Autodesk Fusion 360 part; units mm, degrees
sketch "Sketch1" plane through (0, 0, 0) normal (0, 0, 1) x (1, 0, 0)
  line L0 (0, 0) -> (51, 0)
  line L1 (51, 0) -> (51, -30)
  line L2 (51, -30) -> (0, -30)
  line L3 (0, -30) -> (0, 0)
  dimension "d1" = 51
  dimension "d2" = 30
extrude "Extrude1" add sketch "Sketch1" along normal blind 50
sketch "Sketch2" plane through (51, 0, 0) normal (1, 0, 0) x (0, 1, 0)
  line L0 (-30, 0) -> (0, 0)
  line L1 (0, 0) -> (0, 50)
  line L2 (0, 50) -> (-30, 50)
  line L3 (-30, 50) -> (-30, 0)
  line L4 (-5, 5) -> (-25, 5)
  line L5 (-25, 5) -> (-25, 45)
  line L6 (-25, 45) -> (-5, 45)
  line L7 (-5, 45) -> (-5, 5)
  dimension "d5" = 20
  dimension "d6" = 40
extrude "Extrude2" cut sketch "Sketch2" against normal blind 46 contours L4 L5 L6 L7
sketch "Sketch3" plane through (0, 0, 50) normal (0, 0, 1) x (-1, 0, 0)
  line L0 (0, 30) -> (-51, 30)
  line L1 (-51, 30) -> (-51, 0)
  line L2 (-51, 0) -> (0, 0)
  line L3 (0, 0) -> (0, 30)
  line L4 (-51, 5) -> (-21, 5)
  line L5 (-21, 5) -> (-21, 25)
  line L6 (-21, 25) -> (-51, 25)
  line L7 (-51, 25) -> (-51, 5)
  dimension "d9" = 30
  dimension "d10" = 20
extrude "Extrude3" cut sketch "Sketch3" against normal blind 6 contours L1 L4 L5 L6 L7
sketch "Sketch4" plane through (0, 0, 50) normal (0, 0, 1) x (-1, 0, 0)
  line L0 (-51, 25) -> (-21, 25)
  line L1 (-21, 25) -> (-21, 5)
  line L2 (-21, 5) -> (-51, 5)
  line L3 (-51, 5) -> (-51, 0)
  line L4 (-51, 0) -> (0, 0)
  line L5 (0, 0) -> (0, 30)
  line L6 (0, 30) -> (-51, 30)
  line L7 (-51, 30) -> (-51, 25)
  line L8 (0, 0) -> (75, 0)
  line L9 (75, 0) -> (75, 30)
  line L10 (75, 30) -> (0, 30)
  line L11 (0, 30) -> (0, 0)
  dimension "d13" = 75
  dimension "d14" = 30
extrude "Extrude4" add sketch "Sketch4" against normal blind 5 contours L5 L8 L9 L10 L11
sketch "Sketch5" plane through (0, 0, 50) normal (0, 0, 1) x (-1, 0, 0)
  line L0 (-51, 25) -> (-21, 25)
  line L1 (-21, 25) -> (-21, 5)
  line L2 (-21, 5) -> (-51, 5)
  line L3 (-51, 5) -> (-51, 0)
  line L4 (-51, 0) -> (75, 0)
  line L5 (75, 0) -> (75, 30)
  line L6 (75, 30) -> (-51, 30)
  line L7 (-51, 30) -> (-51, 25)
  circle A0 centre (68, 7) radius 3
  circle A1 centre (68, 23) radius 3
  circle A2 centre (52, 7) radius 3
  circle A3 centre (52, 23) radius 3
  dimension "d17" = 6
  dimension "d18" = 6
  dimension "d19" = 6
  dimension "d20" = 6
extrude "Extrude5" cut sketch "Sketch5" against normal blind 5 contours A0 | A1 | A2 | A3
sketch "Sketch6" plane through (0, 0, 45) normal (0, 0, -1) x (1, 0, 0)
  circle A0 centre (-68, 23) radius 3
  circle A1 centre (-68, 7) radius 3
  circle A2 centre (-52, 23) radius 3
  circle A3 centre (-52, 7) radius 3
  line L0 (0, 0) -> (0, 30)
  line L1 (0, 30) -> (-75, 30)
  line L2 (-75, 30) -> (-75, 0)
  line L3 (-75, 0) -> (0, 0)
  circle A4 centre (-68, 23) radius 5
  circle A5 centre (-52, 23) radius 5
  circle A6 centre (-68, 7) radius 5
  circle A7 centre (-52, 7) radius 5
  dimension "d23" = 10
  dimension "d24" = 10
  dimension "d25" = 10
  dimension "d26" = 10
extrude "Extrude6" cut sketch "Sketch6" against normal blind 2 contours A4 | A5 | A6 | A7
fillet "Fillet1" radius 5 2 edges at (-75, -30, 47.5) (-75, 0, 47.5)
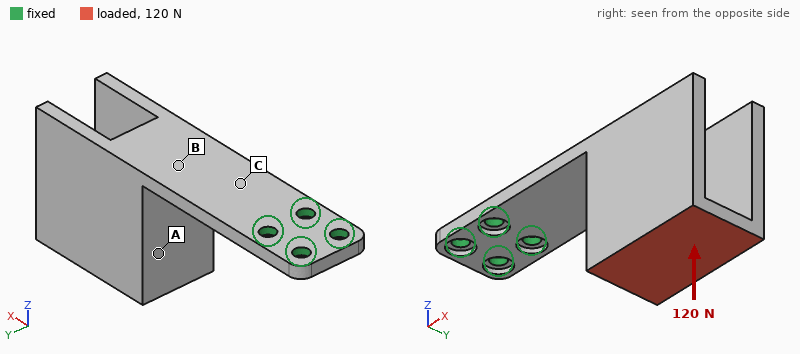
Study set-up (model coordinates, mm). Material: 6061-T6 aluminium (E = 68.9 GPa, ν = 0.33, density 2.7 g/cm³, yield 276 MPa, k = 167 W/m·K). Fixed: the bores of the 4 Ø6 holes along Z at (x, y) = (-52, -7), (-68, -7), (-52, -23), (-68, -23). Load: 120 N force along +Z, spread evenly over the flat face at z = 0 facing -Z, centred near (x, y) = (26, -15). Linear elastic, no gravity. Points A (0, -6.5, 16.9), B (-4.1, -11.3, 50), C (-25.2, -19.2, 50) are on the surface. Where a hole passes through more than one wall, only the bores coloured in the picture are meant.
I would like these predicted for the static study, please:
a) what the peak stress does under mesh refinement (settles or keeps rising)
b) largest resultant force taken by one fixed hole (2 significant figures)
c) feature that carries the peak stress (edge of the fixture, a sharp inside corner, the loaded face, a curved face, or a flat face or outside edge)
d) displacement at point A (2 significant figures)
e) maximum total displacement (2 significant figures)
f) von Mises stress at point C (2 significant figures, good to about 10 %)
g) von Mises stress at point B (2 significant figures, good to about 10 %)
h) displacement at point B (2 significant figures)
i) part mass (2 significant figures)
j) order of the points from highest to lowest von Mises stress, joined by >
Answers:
keeps rising
240 N
edge of the fixture
0.71 mm
1.5 mm
47 MPa
27 MPa
0.44 mm
130 g
C > B > A
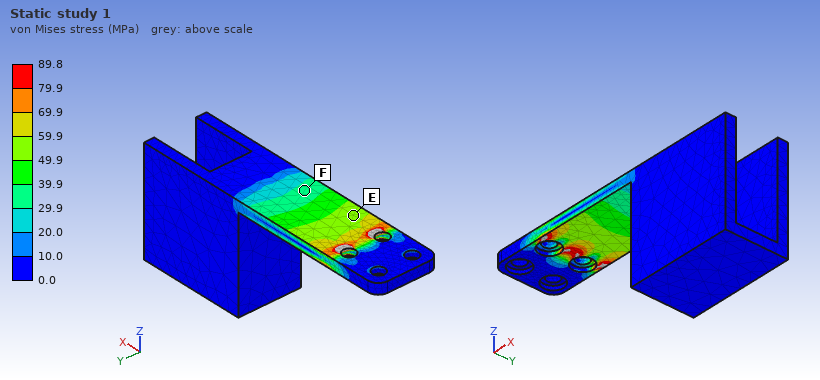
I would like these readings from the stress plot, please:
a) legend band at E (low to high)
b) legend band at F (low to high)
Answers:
49.9 to 59.9 MPa
29.9 to 39.9 MPa
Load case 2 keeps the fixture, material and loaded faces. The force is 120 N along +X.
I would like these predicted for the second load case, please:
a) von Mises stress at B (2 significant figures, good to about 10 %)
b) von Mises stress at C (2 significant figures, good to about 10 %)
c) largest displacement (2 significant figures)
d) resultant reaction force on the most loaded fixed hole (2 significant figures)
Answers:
41 MPa
43 MPa
1.4 mm
140 N
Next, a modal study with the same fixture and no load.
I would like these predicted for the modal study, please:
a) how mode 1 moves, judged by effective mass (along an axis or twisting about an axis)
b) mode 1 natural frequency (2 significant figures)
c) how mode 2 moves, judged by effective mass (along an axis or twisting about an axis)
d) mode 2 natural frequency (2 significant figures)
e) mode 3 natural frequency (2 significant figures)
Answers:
along Z
160 Hz
along Y
410 Hz
1000 Hz
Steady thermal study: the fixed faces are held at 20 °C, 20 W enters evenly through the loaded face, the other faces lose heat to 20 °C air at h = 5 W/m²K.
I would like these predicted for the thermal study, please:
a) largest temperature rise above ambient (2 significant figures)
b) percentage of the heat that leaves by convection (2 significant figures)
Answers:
50 K
17 %
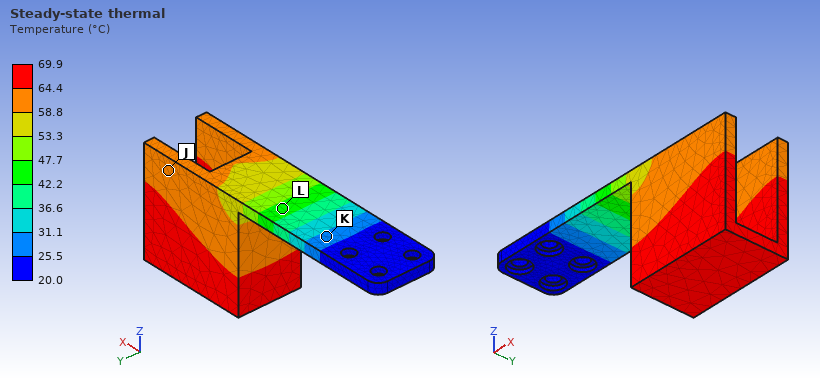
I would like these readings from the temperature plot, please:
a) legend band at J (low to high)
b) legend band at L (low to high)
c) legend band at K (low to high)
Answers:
58.8 to 64.4 °C
42.2 to 47.7 °C
25.5 to 31.1 °C
